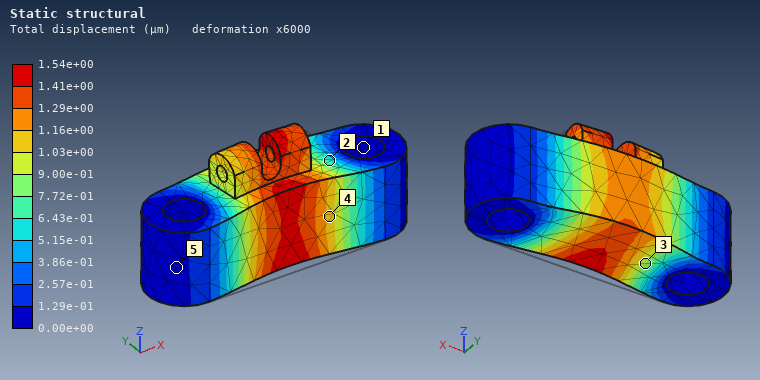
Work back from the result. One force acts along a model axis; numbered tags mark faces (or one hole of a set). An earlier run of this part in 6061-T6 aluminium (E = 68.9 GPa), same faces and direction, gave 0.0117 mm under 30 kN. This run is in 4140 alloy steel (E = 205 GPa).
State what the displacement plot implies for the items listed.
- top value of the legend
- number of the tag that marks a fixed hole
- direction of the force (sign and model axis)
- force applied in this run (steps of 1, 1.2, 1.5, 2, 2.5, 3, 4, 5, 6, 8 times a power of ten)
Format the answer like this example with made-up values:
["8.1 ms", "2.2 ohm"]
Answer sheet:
["1.54e+00 µm", "1", "+Y", "12 kN"]
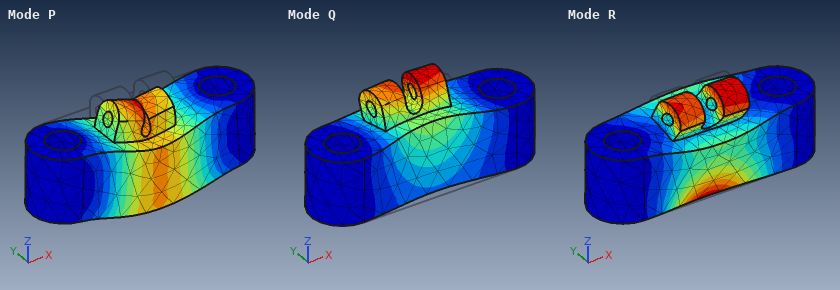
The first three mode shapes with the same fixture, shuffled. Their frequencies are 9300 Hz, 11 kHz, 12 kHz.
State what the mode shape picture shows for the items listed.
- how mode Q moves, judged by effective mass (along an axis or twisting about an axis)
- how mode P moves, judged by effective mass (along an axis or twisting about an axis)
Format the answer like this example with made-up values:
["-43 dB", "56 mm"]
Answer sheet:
["along Y", "along Z"]
